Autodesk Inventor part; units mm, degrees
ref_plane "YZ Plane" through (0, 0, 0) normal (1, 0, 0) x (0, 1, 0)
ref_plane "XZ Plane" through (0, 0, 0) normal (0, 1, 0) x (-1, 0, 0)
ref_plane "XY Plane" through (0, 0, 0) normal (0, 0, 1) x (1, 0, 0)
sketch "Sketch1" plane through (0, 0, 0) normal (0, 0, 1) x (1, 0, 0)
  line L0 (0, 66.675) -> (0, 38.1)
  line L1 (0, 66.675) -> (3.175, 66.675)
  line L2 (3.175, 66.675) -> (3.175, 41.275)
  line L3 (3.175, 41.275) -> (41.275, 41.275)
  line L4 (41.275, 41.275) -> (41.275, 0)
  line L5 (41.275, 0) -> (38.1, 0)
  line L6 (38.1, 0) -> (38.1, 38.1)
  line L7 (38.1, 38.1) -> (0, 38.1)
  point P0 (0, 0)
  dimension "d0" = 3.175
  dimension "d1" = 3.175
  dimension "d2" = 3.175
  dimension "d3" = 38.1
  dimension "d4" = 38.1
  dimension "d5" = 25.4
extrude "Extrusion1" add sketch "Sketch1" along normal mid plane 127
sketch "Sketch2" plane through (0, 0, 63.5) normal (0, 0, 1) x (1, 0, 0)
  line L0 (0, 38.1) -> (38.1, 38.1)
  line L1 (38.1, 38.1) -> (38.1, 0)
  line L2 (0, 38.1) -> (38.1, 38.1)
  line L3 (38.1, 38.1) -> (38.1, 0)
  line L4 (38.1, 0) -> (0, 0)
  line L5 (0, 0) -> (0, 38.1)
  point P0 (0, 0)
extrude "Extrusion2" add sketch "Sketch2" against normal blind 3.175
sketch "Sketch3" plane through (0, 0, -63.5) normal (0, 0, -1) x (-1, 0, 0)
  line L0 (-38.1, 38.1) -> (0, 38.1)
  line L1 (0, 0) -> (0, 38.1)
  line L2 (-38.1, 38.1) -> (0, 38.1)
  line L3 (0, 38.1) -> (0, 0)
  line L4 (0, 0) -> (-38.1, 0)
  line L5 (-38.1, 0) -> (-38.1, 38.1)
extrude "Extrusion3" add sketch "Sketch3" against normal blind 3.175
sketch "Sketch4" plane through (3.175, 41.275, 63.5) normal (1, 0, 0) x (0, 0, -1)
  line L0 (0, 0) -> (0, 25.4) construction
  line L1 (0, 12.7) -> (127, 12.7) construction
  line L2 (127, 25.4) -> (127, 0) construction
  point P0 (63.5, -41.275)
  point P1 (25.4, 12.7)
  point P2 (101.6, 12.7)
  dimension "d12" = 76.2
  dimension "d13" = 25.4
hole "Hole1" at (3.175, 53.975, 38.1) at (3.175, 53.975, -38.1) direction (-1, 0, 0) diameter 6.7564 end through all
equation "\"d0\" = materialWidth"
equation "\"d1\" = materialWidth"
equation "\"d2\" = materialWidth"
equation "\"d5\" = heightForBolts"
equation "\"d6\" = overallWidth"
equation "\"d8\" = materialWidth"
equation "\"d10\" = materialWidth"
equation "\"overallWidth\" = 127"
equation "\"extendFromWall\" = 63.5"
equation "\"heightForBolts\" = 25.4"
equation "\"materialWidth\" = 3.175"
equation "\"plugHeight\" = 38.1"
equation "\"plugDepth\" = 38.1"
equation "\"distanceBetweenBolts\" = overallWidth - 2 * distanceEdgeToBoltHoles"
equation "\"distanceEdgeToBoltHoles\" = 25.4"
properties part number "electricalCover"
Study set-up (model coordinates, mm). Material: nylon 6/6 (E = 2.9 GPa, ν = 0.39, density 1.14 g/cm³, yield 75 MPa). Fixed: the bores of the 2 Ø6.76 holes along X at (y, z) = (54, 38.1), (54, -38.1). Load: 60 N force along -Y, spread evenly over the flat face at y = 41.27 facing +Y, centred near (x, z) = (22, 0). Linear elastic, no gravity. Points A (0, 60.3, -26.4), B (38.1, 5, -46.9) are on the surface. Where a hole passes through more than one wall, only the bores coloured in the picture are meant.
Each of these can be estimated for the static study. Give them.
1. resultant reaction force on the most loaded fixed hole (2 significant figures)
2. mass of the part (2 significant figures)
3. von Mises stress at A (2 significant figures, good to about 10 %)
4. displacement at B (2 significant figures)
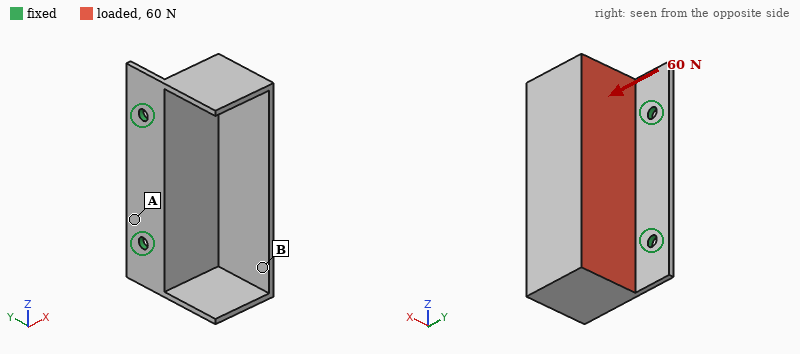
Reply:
30 N
58 g
2.0 MPa
1.5 mm
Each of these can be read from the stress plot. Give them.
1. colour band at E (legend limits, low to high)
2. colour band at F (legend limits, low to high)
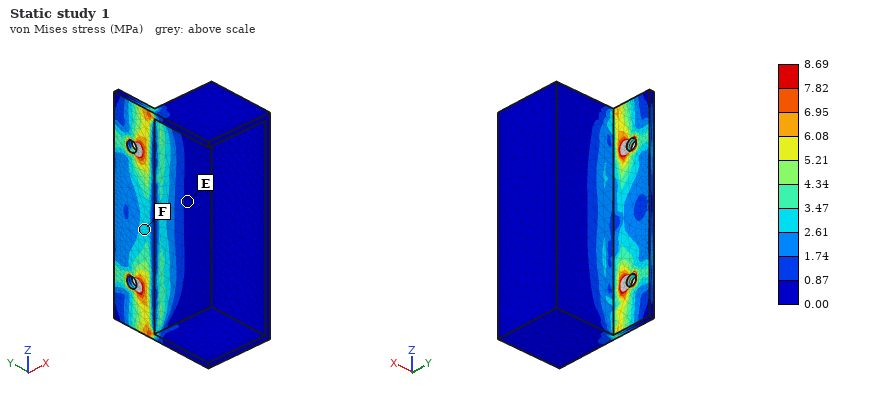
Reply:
0.00 to 0.87 MPa
2.61 to 3.47 MPa
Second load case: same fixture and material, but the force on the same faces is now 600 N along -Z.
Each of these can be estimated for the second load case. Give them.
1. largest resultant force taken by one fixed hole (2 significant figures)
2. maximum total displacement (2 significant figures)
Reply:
350 N
1.7 mm
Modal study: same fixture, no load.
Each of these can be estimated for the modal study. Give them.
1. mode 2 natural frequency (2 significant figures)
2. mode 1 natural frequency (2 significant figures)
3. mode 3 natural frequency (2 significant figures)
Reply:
200 Hz
130 Hz
610 Hz
